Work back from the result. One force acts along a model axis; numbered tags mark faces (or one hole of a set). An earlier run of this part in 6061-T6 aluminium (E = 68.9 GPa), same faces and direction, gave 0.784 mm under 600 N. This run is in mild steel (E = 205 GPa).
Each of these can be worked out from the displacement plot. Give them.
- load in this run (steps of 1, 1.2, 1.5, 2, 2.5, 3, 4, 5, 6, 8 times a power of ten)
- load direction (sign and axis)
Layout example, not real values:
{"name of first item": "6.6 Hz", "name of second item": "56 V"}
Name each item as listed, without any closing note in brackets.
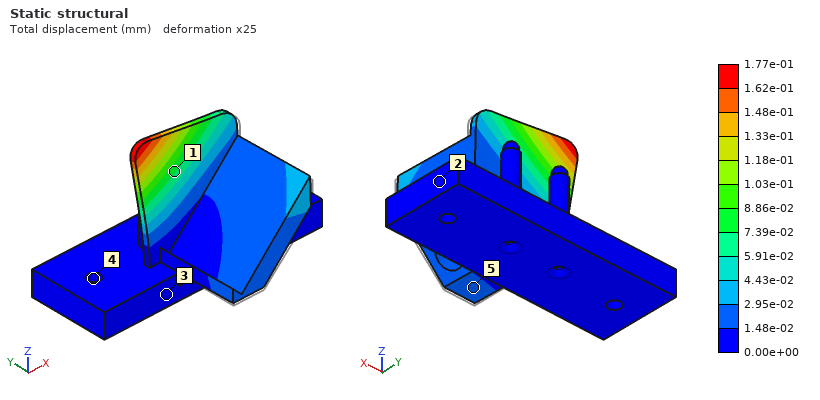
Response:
{"load in this run": "400 N", "load direction": "+Y"}
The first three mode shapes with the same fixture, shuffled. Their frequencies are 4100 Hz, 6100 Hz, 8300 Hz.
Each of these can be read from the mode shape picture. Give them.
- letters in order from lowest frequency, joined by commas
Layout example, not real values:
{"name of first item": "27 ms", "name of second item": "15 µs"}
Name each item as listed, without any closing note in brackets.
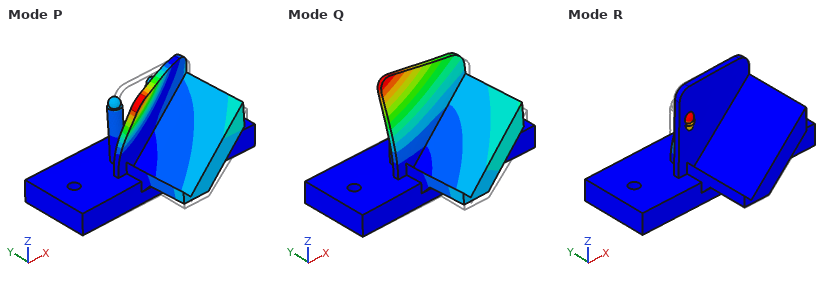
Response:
{"letters in order from lowest frequency, joined by commas": "Q, P, R"}
